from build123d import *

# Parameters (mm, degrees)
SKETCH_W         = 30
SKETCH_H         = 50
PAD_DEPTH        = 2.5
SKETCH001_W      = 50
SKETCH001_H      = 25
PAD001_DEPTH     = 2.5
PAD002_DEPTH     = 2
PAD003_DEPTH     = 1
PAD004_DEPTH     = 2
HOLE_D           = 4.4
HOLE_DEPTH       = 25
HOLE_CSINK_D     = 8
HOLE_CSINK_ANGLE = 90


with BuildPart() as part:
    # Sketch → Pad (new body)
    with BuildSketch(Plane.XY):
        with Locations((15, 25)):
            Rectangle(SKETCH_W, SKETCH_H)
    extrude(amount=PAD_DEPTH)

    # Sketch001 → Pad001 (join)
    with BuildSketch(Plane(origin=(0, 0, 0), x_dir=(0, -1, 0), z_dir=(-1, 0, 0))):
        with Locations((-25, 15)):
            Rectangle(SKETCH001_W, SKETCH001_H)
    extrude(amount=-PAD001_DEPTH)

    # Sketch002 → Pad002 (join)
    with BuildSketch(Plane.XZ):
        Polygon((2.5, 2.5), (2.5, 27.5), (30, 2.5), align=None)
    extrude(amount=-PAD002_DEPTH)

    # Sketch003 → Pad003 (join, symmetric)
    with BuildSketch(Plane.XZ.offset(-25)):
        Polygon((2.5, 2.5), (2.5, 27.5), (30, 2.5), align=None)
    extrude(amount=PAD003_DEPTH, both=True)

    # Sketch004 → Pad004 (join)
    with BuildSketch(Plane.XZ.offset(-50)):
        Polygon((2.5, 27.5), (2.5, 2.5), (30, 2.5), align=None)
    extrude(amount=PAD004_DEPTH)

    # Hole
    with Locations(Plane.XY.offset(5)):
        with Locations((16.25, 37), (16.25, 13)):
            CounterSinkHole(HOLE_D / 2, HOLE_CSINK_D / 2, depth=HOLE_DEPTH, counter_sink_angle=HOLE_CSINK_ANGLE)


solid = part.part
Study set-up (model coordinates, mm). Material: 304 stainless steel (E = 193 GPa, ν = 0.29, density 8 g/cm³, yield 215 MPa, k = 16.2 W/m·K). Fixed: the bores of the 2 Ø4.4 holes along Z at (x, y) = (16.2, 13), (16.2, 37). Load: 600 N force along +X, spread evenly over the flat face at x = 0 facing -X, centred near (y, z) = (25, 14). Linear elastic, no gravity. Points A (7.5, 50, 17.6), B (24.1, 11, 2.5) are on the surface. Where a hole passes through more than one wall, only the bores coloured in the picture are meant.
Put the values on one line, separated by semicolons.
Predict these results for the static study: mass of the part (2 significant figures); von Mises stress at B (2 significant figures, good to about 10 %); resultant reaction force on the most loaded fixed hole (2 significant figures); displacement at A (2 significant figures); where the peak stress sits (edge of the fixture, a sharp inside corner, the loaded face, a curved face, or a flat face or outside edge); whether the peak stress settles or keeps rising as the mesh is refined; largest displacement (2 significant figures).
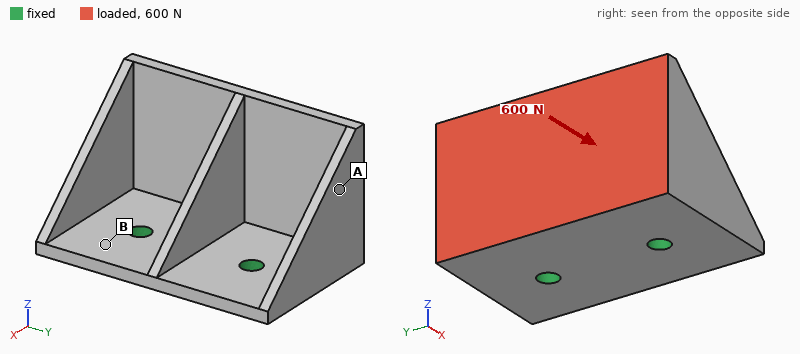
71 g; 36 MPa; 300 N; 32 µm; edge of the fixture; keeps rising; 56 µm
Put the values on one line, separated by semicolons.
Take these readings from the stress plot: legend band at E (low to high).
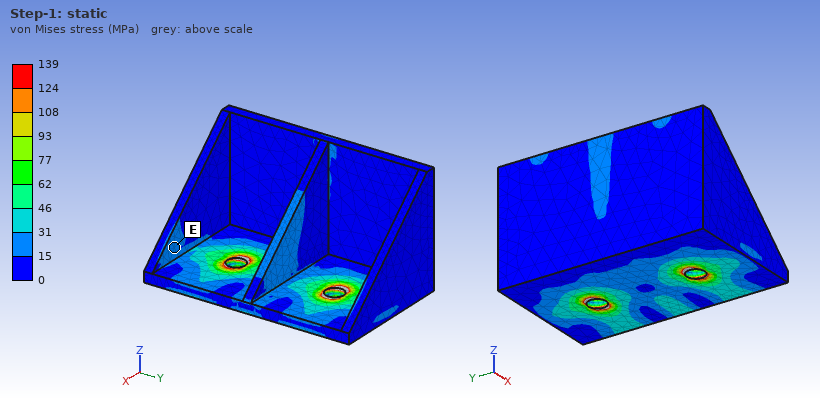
15 to 31 MPa
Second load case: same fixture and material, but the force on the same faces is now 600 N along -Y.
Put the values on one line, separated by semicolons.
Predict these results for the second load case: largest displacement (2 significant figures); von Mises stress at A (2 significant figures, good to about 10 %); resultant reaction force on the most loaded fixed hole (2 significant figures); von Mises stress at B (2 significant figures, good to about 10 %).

45 µm; 10 MPa; 520 N; 12 MPa
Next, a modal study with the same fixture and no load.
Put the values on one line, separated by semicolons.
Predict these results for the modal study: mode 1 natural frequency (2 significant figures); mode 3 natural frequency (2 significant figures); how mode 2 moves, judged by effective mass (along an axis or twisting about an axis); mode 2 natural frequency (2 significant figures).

2600 Hz; 6100 Hz; along Y; 2800 Hz
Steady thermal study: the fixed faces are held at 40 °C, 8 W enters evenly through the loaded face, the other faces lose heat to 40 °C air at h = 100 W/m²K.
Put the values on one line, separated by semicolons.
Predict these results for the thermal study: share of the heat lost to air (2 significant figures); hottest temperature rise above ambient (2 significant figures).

81 %; 25 K
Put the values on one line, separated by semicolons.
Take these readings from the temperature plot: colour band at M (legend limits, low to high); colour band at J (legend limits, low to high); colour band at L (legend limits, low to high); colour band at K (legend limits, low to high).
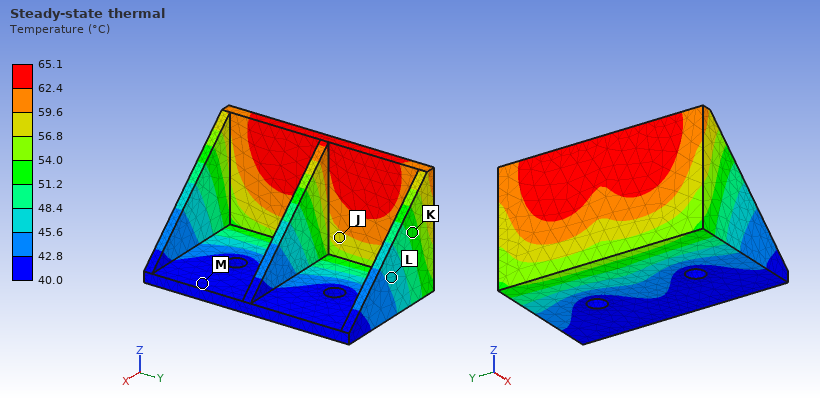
40.0 to 42.8 °C; 56.8 to 59.6 °C; 45.6 to 48.4 °C; 51.2 to 54.0 °C
